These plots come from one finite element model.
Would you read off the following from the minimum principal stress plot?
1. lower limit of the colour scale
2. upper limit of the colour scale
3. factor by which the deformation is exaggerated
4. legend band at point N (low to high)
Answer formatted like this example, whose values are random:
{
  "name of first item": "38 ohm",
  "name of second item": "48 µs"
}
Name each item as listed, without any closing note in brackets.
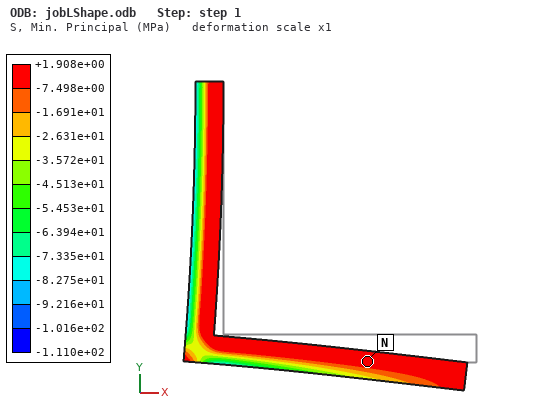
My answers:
{
  "lower limit of the colour scale": "-1.110e+02 MPa",
  "upper limit of the colour scale": "+1.908e+00 MPa",
  "factor by which the deformation is exaggerated": "1",
  "legend band at point N": "-7.498e+00 to +1.908e+00 MPa"
}
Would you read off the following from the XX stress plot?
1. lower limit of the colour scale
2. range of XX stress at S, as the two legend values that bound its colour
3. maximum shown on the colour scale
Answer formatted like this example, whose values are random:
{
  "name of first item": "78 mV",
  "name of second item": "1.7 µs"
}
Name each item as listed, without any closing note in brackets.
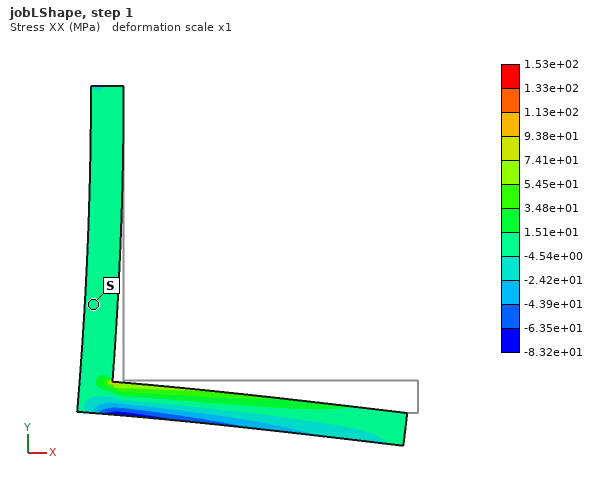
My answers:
{
  "lower limit of the colour scale": "-8.32e+01 MPa",
  "range of XX stress at S, as the two legend values that bound its colour": "-4.54e+00 to 1.51e+01 MPa",
  "maximum shown on the colour scale": "1.53e+02 MPa"
}
